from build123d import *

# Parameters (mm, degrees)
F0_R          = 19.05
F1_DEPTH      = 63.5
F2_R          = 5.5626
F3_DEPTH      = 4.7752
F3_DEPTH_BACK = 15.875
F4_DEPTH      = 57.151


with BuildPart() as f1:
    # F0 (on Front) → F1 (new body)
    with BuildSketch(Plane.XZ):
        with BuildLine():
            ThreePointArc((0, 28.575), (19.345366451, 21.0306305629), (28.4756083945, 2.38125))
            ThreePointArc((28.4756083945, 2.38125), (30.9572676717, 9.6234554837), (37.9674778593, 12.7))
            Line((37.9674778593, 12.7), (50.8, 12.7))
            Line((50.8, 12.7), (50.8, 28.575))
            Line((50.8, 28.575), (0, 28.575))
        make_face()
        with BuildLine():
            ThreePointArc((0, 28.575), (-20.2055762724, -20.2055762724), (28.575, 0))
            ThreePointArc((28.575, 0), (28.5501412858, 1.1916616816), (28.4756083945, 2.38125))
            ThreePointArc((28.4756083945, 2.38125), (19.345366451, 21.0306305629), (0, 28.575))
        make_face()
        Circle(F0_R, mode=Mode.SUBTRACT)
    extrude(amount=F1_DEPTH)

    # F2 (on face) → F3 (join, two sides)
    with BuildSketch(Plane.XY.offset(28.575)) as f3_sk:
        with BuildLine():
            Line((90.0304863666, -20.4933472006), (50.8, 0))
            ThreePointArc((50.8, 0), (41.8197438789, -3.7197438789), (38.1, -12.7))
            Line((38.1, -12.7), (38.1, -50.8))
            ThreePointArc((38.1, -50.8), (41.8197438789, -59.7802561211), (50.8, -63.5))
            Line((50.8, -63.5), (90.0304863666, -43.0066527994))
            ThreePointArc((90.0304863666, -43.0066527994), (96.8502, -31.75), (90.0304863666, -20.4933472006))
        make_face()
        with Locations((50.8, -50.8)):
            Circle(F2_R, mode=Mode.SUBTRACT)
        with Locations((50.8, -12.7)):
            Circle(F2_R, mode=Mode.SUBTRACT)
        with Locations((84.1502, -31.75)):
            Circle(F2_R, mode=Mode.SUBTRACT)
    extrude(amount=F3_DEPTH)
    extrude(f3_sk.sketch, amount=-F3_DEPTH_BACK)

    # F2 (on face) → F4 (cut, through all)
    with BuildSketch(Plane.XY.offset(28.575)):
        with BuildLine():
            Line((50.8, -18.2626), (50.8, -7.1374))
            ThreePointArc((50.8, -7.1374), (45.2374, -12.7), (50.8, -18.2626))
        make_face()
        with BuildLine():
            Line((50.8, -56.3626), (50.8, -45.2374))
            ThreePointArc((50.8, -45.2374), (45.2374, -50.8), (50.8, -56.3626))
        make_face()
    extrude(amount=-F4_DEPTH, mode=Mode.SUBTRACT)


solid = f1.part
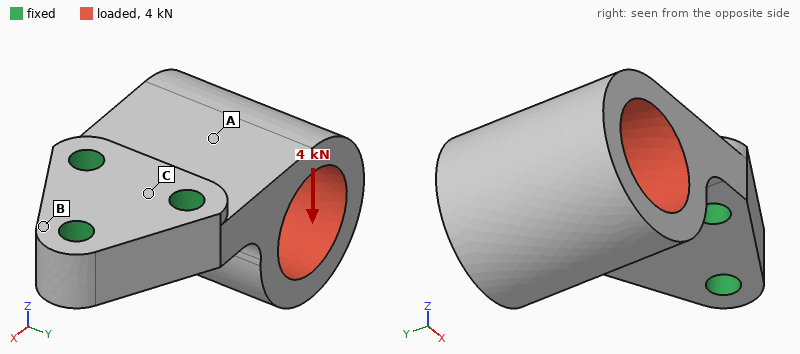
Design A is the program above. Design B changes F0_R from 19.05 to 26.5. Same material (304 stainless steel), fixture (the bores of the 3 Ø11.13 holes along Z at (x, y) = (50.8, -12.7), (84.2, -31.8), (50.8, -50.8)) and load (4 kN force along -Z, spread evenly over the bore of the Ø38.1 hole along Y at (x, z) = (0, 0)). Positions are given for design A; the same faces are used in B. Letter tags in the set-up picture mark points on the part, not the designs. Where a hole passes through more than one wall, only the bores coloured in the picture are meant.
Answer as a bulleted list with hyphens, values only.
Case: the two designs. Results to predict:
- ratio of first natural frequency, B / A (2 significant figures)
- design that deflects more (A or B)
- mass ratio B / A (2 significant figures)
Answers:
- 0.44
- B
- 0.58
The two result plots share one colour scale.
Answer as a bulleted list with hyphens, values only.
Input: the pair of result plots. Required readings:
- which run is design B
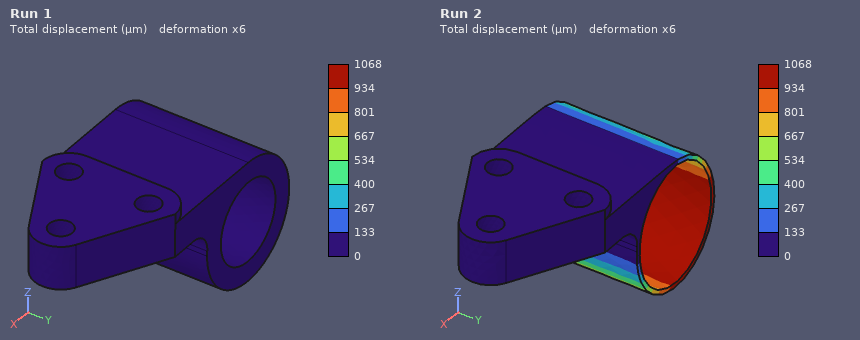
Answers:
- Run 2
